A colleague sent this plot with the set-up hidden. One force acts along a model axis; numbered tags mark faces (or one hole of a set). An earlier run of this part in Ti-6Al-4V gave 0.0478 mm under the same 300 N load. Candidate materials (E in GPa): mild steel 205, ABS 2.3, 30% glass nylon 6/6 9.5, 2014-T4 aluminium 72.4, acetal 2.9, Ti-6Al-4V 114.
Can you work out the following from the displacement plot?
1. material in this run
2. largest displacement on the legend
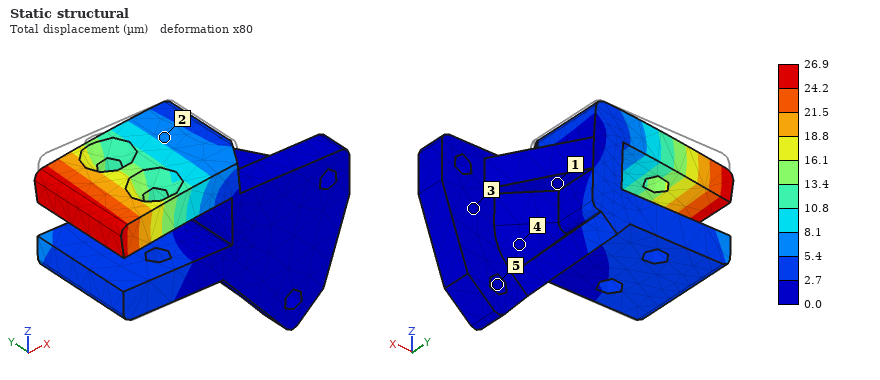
mild steel
26.9 µm
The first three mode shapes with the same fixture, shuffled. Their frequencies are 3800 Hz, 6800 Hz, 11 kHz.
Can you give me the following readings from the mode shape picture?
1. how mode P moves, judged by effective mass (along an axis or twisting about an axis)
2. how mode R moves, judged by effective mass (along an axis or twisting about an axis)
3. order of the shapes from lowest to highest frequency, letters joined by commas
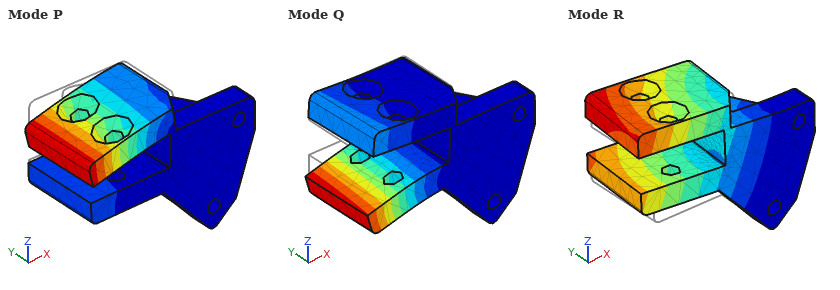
along Z
along Y
R, P, Q
